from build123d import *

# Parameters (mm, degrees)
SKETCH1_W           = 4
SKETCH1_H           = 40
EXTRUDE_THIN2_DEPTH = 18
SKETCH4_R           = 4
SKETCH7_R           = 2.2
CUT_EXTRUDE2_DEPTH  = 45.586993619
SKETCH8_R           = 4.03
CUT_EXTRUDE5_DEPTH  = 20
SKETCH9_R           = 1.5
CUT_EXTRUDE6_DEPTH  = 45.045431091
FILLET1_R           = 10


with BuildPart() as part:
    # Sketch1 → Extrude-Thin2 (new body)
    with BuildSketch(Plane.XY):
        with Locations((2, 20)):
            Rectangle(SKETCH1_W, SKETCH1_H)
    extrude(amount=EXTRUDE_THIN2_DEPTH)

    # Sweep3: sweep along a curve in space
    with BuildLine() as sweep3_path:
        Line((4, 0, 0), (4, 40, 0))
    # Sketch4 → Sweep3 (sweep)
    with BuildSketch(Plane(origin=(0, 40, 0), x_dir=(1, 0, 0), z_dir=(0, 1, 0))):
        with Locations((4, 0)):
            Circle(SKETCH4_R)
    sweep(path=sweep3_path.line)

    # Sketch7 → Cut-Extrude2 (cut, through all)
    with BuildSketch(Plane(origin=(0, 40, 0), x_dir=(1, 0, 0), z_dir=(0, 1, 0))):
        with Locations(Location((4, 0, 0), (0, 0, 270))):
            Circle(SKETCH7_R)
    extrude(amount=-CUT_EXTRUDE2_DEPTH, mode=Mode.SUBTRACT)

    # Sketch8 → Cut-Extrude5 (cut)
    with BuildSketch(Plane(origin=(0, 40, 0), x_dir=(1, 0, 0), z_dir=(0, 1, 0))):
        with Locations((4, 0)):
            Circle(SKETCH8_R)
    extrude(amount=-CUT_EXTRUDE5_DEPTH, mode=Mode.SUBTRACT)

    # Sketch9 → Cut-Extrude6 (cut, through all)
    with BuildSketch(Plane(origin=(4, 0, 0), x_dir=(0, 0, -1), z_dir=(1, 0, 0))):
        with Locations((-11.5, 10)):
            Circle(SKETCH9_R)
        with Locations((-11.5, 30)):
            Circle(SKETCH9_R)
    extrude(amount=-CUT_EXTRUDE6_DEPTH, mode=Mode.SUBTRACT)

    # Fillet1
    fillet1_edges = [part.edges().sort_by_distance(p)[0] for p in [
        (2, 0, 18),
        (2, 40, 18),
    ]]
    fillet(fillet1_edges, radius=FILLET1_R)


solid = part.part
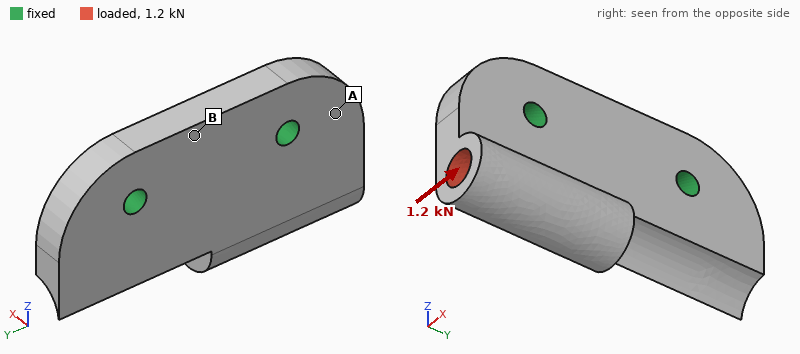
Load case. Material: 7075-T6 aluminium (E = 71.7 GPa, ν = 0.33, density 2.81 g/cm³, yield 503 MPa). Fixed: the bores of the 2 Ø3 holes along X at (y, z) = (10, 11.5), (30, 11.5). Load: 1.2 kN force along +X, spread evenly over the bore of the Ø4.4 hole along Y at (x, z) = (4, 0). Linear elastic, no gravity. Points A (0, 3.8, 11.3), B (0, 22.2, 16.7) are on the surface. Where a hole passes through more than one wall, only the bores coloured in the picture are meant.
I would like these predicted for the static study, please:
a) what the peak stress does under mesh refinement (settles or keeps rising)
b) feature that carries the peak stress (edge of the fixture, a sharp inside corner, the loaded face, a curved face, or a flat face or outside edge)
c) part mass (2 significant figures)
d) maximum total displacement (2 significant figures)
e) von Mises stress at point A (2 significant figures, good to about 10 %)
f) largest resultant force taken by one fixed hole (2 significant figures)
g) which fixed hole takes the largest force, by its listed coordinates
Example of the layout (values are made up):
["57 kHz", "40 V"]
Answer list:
["keeps rising", "edge of the fixture", "8.0 g", "0.16 mm", "100 MPa", "1.1 kN", "(10, 11.5)"]
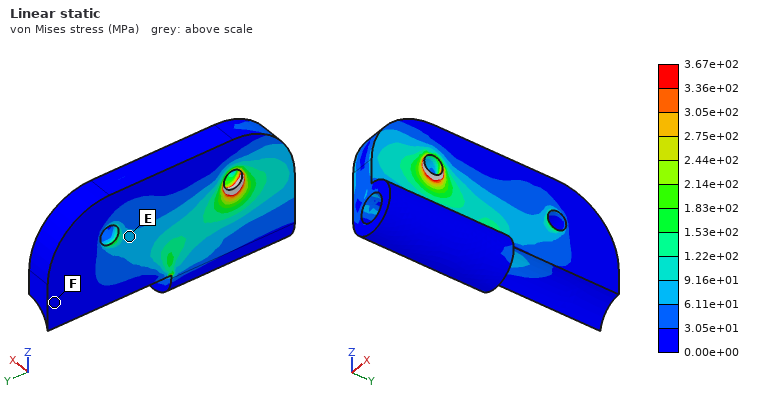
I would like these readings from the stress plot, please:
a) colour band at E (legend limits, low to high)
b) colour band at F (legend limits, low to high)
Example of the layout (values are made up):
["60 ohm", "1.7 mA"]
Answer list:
["6.11e+01 to 9.16e+01 MPa", "0.00e+00 to 3.05e+01 MPa"]
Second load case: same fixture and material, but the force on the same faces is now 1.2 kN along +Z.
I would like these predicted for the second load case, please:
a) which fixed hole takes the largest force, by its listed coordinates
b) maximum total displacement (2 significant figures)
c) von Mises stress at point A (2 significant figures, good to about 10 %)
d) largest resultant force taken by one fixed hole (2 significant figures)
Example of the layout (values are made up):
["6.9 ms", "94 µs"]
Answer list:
["(10, 11.5)", "41 µm", "13 MPa", "1.2 kN"]
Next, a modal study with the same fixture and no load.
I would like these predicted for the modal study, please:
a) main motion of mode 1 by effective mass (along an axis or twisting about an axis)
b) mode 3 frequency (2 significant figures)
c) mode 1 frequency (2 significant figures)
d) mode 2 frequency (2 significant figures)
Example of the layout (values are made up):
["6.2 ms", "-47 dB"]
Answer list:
["along X", "28 kHz", "11 kHz", "20 kHz"]
